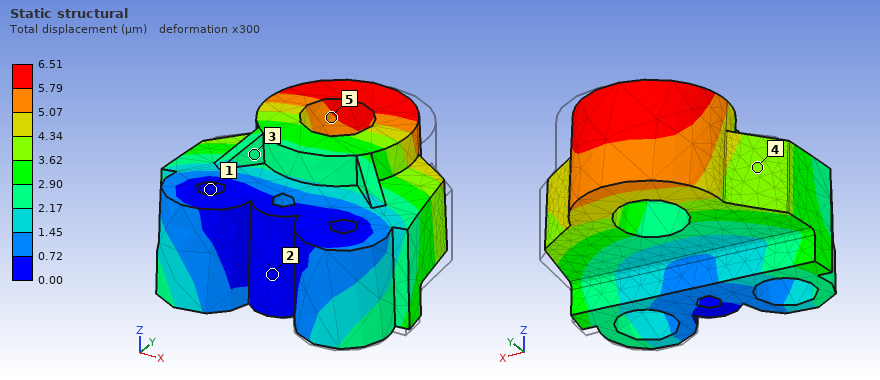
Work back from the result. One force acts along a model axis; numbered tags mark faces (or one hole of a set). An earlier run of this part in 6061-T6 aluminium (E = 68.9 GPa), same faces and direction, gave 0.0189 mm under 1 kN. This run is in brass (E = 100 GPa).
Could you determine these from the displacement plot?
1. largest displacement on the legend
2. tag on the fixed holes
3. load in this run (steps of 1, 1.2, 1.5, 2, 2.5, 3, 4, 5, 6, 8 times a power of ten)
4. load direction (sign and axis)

6.51 µm
1
500 N
-X
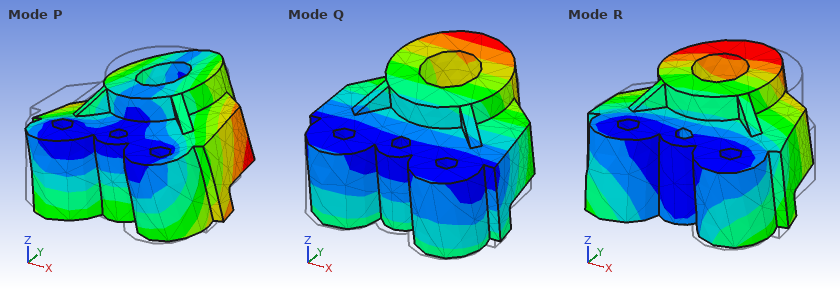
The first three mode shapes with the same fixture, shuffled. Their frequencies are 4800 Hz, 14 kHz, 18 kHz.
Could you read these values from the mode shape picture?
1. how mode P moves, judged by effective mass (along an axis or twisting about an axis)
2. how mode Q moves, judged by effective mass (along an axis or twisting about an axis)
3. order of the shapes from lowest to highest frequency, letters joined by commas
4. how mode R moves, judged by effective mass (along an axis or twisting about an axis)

along X
along Z
Q, R, P
along X
